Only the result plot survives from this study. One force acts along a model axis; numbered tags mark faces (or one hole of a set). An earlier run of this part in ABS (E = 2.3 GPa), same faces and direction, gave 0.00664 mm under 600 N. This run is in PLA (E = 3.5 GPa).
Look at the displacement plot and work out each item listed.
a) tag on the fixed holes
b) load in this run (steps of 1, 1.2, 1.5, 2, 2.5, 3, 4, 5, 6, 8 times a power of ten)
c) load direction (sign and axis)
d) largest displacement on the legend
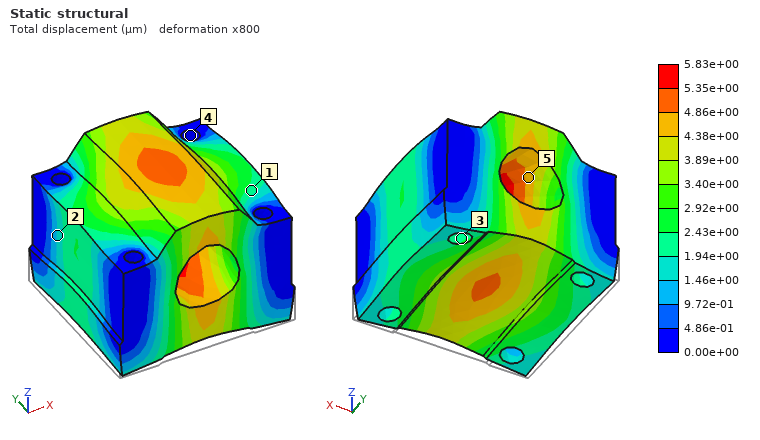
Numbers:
4
800 N
+Z
5.83e+00 µm
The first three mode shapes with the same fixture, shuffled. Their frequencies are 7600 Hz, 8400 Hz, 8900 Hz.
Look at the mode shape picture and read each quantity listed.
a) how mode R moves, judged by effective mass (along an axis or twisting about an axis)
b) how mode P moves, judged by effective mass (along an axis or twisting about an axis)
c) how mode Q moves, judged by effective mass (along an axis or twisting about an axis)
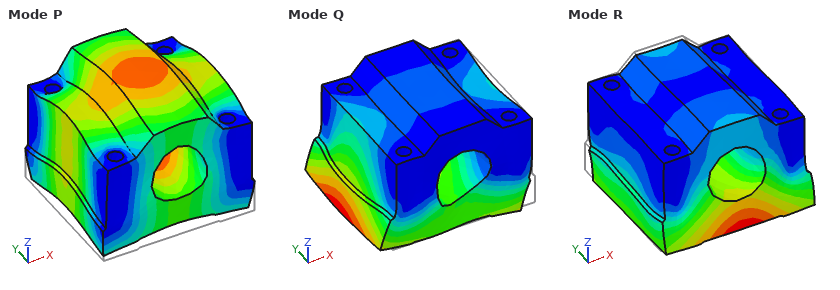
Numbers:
along Y
along Z
along X
